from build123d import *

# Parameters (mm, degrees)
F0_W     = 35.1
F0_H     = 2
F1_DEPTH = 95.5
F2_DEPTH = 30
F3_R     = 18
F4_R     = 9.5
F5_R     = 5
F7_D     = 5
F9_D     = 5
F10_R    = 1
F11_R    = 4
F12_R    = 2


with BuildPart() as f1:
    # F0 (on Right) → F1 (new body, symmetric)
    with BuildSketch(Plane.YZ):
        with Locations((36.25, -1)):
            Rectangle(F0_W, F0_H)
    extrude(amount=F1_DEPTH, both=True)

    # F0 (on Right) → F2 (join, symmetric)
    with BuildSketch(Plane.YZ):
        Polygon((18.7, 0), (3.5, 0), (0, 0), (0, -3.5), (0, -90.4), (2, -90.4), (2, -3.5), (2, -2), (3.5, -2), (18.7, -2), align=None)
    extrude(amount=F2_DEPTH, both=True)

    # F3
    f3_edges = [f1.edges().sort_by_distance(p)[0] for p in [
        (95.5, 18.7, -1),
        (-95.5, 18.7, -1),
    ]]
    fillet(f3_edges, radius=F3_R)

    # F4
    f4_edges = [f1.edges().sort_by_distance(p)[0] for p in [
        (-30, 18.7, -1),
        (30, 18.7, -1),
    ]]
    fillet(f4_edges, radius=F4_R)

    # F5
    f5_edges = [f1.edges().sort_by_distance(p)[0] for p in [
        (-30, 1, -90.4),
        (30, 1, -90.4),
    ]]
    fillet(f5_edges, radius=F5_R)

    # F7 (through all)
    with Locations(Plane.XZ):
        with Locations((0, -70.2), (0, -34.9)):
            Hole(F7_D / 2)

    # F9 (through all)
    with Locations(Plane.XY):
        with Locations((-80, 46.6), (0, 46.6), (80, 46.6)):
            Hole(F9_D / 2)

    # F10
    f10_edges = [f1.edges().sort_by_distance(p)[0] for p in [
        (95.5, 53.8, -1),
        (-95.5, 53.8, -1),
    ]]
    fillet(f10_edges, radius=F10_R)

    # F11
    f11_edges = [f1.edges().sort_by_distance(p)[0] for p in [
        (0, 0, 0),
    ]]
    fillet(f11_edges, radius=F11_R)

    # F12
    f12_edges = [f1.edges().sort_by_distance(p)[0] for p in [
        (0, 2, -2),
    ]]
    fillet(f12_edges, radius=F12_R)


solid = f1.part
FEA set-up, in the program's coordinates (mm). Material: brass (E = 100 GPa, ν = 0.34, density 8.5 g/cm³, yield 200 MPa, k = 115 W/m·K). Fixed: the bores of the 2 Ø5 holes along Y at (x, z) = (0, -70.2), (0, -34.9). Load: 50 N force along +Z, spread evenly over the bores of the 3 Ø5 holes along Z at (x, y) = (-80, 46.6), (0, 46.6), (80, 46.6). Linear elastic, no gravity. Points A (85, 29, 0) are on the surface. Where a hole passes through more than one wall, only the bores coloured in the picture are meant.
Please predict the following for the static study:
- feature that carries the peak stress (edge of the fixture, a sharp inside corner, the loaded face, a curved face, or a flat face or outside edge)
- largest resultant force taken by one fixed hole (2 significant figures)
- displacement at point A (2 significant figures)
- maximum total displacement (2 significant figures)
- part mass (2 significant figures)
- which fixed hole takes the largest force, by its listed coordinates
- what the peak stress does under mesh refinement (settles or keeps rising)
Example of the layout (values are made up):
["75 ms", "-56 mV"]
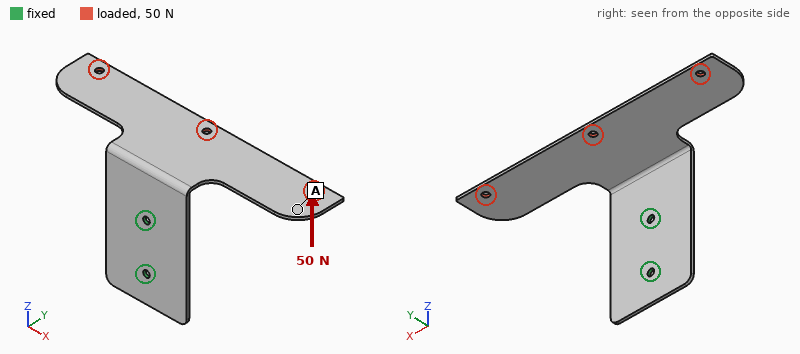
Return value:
["edge of the fixture", "45 N", "1.4 mm", "2.3 mm", "220 g", "(0, -34.9)", "keeps rising"]
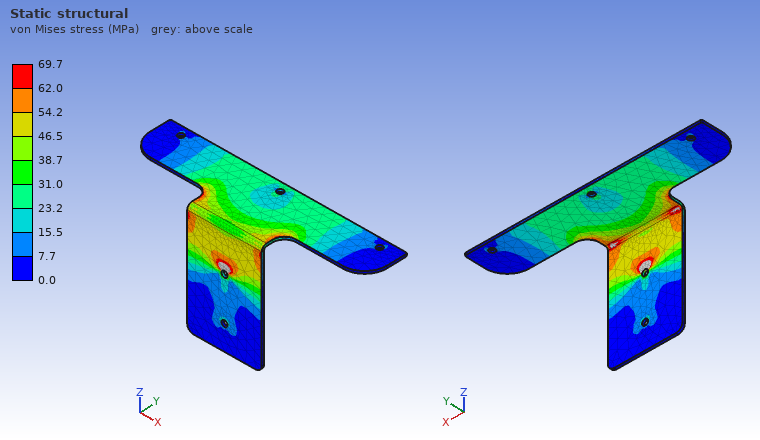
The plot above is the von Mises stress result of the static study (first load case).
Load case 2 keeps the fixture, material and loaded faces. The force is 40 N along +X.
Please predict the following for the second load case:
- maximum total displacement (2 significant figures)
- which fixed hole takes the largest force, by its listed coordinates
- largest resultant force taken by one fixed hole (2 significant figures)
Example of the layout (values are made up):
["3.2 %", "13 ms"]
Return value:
["1.0 mm", "(0, -34.9)", "74 N"]
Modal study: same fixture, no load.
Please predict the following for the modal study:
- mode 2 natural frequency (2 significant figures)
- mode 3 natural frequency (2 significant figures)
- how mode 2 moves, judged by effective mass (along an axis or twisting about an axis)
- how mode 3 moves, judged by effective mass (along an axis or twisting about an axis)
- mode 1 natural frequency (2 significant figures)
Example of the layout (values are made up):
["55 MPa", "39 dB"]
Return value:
["100 Hz", "140 Hz", "along Z", "twisting about Y", "99 Hz"]
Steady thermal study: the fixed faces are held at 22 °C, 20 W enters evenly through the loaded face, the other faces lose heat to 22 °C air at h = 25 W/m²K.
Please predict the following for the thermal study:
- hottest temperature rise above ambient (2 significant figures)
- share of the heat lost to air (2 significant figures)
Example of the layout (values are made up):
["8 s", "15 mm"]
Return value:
["60 K", "77 %"]
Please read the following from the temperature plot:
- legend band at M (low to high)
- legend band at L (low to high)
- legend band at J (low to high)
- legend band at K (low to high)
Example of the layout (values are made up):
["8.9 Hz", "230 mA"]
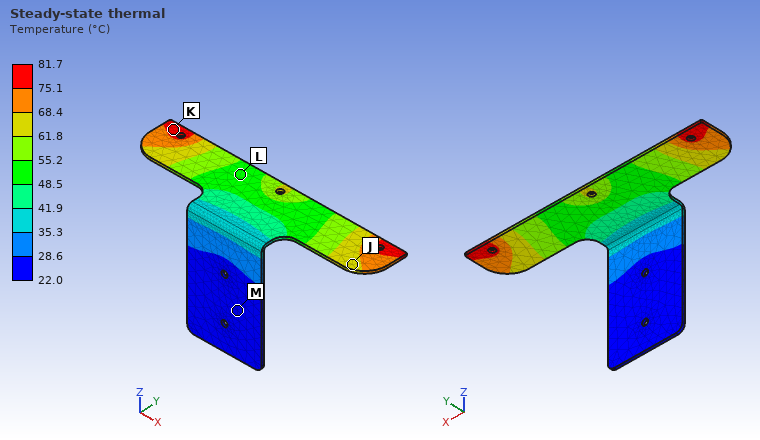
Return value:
["22.0 to 28.6 °C", "48.5 to 55.2 °C", "61.8 to 68.4 °C", "75.1 to 81.7 °C"]
